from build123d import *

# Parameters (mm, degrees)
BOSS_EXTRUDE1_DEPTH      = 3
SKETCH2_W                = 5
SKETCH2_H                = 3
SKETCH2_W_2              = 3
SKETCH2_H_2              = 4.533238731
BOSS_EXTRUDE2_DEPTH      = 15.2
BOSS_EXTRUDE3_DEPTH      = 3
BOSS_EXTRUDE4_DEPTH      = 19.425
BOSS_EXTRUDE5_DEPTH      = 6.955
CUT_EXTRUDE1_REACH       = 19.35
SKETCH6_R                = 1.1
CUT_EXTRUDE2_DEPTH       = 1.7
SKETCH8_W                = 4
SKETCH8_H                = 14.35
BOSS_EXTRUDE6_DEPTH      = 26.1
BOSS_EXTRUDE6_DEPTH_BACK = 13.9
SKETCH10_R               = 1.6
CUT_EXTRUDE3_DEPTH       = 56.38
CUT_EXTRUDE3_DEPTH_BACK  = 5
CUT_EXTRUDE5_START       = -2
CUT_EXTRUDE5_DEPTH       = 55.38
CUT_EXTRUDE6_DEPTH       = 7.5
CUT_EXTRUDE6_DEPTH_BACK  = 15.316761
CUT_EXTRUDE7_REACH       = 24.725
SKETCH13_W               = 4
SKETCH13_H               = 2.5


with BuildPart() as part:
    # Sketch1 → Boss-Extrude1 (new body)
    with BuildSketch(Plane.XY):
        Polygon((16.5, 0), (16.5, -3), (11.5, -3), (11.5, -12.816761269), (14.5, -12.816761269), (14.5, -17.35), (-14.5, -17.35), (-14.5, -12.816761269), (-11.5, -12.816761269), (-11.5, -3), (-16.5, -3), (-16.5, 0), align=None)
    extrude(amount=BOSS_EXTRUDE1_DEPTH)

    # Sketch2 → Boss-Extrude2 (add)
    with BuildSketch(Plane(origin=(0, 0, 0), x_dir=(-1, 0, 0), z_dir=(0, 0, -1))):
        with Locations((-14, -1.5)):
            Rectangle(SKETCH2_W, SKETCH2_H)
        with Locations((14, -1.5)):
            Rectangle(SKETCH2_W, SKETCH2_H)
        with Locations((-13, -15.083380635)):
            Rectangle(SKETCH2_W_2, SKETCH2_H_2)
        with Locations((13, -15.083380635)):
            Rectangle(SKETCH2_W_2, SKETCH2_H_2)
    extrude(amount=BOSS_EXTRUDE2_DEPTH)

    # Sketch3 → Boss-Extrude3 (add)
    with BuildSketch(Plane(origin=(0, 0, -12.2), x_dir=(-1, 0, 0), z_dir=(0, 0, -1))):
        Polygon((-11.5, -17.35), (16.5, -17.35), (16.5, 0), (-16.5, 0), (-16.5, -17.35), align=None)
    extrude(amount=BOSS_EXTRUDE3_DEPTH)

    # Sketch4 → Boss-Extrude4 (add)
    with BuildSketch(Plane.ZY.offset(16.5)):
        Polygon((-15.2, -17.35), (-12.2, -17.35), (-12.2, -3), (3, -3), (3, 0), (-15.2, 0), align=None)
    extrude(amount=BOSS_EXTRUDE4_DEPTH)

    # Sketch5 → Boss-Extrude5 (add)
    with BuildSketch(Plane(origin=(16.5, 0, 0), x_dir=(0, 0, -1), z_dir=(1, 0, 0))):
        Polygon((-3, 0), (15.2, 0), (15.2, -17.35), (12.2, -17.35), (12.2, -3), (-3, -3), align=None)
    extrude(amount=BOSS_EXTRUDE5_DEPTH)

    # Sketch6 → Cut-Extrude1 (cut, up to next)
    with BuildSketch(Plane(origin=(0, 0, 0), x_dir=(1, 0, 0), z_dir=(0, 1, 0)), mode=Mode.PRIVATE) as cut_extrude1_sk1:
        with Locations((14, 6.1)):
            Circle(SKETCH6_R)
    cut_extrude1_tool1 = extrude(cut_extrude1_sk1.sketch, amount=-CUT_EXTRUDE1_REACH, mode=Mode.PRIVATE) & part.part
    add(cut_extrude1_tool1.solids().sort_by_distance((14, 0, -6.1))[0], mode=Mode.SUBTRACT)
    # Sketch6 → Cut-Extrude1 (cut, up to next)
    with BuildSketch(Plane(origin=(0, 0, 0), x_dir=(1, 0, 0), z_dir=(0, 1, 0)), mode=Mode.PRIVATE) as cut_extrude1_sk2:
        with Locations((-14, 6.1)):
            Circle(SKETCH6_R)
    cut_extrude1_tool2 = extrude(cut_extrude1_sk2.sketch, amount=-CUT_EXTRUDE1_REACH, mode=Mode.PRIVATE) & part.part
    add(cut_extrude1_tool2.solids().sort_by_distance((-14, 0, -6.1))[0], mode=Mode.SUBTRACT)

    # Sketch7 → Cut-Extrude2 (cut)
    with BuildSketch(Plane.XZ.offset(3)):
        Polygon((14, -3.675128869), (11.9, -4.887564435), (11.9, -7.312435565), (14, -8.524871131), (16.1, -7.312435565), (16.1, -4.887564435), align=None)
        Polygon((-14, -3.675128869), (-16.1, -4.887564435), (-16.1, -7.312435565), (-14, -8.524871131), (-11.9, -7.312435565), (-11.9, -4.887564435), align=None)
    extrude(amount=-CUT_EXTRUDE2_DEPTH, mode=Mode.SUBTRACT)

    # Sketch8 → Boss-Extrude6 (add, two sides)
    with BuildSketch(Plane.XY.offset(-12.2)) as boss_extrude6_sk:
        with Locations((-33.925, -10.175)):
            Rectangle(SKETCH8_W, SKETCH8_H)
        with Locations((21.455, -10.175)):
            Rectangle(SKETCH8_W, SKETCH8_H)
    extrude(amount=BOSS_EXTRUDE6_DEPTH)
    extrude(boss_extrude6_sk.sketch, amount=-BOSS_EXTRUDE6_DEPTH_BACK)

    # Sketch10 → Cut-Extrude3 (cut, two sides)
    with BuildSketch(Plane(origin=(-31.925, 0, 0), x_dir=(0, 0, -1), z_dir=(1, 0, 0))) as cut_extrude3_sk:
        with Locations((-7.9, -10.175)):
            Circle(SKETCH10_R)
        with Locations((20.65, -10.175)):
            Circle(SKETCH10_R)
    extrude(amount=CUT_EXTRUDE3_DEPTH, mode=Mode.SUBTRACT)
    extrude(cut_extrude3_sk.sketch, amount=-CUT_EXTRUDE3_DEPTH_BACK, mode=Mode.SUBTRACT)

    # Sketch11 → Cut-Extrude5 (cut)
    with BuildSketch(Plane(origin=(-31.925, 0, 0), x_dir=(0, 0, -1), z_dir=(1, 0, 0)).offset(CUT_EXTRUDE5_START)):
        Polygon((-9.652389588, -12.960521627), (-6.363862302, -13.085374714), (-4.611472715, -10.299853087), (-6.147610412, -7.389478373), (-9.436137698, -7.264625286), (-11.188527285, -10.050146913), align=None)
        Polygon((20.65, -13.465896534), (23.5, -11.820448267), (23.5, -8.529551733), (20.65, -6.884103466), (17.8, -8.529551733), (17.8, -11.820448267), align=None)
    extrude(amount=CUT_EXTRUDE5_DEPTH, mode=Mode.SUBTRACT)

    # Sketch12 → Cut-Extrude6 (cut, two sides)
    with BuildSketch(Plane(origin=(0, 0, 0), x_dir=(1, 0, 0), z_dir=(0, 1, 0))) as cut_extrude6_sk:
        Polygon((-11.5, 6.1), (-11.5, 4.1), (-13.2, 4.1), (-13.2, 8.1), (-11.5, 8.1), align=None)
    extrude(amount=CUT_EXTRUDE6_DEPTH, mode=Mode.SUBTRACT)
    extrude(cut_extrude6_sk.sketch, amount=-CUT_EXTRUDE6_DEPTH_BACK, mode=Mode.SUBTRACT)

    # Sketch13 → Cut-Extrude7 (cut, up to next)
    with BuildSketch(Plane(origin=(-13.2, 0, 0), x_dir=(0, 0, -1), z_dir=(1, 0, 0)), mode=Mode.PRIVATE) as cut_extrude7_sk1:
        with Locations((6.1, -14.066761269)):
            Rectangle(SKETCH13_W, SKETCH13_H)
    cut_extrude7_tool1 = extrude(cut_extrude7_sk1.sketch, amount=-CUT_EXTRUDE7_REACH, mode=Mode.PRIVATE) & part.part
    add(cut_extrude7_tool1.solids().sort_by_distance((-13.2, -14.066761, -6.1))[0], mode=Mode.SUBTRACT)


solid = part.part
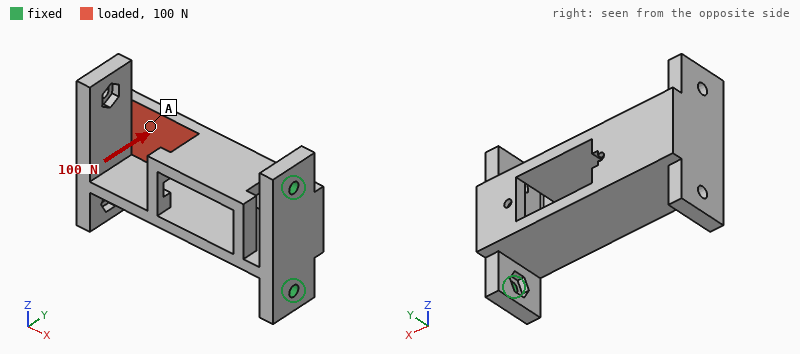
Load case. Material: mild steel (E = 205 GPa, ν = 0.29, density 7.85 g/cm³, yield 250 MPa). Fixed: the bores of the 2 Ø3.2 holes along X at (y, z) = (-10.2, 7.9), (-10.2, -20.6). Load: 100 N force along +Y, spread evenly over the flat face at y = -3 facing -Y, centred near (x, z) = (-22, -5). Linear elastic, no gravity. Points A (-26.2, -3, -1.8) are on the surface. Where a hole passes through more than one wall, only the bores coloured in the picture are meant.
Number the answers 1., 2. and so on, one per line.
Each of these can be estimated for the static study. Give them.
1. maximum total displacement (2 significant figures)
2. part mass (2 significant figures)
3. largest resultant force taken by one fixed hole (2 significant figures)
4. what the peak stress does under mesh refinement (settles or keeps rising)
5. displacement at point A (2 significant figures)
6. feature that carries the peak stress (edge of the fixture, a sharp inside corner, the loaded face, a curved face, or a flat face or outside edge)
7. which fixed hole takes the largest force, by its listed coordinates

1. 0.12 mm
2. 80 g
3. 61 N
4. keeps rising
5. 0.095 mm
6. edge of the fixture
7. (-10.2, 7.9)
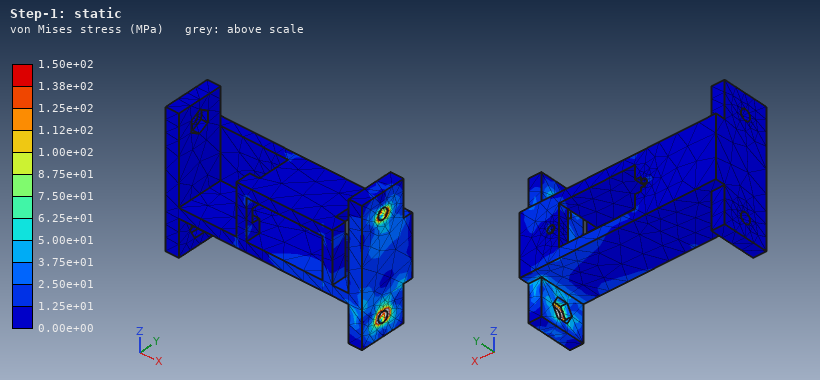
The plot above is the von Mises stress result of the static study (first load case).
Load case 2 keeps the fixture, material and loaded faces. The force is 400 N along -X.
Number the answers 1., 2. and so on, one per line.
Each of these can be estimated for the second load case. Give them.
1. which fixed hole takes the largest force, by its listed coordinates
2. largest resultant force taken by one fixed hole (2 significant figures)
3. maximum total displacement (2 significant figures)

1. (-10.2, 7.9)
2. 280 N
3. 53 µm
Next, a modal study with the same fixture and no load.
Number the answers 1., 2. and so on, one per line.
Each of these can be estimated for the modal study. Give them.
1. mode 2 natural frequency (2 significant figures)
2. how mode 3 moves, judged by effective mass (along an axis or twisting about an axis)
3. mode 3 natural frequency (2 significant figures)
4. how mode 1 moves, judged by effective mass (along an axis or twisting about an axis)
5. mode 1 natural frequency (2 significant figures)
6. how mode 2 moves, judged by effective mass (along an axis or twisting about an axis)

1. 1200 Hz
2. twisting about X
3. 2600 Hz
4. along Y
5. 750 Hz
6. along Z
